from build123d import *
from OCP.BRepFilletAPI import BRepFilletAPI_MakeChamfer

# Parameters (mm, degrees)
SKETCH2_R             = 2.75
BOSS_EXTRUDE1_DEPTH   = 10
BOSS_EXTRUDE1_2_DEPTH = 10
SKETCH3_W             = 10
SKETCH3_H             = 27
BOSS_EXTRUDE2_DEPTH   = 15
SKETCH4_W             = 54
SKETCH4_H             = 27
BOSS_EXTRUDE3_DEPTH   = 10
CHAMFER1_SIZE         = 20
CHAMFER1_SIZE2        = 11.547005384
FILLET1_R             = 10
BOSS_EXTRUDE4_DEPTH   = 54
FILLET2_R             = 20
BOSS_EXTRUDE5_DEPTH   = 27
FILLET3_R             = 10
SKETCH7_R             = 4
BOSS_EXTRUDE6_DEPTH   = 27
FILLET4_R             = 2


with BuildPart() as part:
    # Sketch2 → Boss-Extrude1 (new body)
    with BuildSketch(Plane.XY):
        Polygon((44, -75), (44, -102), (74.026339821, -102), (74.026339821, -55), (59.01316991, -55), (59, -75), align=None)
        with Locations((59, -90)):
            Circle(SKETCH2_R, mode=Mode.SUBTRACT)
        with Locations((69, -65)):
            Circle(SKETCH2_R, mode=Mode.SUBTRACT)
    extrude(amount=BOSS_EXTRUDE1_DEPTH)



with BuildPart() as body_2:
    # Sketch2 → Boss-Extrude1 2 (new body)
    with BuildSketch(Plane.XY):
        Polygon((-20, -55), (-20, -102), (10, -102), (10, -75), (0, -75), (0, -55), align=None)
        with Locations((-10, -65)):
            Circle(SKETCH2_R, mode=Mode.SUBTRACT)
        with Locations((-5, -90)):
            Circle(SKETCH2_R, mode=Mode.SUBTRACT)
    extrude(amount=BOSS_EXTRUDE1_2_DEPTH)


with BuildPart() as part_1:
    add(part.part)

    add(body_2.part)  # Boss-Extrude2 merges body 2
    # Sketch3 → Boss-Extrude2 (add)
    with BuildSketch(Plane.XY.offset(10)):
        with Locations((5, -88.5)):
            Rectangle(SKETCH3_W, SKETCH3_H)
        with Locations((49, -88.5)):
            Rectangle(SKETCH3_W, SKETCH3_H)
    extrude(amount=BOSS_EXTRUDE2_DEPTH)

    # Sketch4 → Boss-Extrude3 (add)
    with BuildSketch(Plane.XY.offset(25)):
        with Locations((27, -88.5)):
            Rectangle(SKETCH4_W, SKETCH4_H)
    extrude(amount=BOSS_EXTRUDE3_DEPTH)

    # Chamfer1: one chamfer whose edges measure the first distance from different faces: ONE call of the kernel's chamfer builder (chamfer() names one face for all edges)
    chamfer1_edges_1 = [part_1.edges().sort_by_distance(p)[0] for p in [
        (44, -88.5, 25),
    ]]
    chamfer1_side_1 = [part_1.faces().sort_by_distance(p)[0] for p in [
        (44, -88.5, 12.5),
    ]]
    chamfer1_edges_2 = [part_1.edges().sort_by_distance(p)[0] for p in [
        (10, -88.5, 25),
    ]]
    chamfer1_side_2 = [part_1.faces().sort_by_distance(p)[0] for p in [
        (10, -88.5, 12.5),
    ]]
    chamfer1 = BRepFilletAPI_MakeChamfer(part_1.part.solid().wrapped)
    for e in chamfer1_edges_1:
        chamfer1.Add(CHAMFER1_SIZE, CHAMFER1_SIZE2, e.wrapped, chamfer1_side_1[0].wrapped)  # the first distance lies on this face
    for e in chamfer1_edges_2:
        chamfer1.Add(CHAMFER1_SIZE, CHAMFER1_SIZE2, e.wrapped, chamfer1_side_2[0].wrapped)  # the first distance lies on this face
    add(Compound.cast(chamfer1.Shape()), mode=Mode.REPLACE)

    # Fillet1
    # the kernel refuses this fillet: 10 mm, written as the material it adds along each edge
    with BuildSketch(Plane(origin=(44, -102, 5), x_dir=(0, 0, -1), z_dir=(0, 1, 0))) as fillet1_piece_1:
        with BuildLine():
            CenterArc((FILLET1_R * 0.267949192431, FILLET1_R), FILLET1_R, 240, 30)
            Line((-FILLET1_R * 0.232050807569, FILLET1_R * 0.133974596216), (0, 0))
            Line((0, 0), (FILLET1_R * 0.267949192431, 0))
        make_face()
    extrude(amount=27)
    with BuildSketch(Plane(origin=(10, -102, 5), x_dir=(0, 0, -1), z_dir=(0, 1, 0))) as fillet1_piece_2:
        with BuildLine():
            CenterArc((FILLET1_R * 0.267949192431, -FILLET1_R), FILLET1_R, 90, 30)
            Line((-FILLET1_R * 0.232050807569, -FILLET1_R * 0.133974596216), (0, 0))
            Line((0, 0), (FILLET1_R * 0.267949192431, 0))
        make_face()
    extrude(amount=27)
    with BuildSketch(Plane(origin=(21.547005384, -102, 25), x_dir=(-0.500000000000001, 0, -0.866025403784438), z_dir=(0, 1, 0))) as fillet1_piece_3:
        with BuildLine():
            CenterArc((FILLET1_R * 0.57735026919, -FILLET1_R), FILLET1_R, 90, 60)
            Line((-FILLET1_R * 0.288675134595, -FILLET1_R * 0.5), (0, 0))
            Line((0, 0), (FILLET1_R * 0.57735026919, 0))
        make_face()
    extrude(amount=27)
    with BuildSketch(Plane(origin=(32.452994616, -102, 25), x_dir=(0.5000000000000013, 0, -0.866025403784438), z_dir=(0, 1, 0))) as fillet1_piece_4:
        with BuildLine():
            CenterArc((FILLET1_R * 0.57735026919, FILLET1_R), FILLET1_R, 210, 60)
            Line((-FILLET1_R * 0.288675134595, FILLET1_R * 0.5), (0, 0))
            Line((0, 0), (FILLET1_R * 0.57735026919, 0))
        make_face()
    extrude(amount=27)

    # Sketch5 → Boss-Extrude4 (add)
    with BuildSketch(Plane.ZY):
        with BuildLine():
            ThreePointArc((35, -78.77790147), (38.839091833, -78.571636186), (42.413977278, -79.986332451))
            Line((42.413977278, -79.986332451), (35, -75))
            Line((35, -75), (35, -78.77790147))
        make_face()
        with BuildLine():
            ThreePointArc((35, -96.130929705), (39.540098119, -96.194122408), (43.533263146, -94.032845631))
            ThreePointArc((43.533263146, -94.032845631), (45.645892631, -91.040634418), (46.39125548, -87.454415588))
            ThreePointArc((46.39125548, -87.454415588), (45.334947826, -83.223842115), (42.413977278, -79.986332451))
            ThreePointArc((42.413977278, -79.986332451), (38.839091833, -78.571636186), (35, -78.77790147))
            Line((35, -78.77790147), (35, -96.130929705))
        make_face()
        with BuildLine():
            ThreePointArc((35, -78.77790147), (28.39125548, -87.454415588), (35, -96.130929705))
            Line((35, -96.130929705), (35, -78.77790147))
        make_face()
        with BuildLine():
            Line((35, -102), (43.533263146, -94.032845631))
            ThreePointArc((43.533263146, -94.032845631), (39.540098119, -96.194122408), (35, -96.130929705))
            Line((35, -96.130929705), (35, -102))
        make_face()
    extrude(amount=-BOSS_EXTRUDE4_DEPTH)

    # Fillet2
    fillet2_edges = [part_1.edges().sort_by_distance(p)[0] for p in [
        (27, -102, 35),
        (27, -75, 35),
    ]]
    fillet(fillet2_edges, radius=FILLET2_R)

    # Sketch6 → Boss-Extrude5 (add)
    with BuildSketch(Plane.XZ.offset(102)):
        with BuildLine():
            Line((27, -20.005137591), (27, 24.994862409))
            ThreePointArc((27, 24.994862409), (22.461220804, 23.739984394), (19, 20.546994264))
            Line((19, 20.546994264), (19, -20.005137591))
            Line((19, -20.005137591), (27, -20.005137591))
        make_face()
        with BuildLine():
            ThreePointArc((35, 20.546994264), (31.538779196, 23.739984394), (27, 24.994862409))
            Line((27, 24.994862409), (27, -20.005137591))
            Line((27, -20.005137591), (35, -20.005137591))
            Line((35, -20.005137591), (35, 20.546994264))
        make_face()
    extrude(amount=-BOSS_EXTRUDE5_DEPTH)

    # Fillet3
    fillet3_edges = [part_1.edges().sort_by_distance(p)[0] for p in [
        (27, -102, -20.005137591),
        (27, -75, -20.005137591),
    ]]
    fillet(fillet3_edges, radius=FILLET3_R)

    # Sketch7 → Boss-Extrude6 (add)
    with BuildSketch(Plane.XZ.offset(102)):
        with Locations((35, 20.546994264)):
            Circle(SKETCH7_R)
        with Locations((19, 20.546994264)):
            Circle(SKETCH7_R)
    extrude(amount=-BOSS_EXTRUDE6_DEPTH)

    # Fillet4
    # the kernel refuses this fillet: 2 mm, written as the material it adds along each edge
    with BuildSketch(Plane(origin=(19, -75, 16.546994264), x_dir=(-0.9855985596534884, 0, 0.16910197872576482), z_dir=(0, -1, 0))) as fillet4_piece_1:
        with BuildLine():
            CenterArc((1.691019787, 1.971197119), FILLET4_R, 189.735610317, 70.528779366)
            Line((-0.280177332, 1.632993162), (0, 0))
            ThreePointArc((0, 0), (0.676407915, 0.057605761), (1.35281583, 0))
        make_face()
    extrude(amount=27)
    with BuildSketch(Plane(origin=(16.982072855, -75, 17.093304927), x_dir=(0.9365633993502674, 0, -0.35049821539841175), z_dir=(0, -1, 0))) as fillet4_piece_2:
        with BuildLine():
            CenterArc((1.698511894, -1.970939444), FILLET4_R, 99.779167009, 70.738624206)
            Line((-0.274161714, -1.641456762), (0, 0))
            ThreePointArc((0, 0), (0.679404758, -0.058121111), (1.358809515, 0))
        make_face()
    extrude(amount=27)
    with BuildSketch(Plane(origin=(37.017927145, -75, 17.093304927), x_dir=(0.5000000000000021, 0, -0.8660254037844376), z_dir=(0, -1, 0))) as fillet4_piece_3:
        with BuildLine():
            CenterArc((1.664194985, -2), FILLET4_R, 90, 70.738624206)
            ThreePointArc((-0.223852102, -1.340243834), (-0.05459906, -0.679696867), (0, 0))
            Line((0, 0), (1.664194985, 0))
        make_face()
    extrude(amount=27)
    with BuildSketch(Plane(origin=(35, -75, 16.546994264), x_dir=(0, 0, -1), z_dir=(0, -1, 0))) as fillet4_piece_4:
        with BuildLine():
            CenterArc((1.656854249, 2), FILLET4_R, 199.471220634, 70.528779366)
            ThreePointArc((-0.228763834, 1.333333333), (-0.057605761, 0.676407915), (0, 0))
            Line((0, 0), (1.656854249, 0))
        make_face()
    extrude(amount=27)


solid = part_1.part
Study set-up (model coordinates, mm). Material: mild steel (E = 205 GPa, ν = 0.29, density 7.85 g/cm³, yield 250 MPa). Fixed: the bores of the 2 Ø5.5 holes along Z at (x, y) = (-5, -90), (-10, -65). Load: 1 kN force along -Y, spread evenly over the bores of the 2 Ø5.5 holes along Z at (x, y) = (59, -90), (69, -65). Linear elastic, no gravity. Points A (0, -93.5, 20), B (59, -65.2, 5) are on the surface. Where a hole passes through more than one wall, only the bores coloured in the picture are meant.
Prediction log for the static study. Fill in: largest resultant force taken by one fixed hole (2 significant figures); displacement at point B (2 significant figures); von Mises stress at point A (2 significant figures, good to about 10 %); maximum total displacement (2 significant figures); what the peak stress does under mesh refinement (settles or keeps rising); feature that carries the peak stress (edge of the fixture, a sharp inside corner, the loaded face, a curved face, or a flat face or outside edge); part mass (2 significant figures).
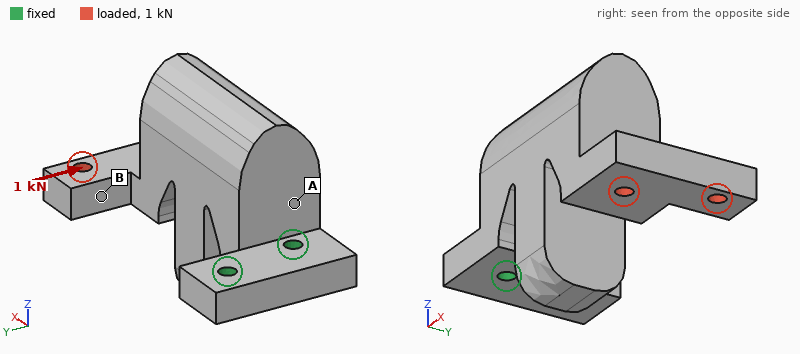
2.4 kN
68 µm
35 MPa
92 µm
keeps rising
edge of the fixture
630 g
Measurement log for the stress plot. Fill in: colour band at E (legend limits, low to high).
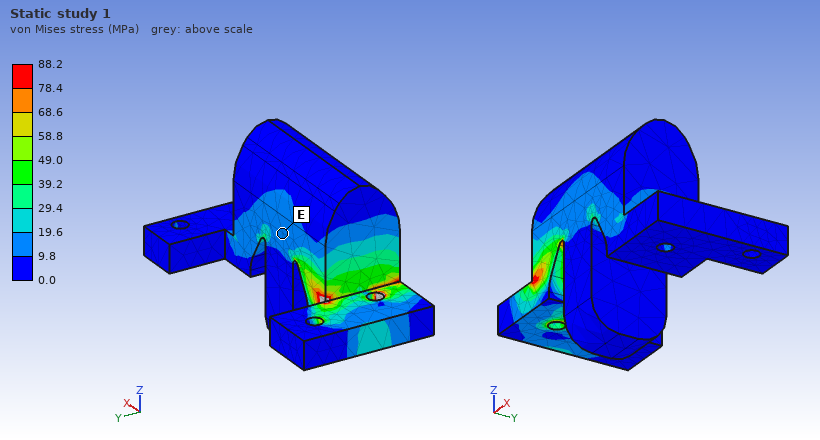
9.8 to 19.6 MPa
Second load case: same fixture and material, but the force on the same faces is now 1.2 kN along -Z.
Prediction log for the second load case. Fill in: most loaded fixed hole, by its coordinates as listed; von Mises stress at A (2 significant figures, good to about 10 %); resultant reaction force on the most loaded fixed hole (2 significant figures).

(-5, -90)
45 MPa
1.3 kN
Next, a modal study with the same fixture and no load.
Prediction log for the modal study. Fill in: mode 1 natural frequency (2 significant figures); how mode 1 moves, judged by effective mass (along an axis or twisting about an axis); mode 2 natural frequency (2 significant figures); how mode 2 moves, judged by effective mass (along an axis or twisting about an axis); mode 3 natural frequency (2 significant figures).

900 Hz
along Z
1500 Hz
along Y
2800 Hz
